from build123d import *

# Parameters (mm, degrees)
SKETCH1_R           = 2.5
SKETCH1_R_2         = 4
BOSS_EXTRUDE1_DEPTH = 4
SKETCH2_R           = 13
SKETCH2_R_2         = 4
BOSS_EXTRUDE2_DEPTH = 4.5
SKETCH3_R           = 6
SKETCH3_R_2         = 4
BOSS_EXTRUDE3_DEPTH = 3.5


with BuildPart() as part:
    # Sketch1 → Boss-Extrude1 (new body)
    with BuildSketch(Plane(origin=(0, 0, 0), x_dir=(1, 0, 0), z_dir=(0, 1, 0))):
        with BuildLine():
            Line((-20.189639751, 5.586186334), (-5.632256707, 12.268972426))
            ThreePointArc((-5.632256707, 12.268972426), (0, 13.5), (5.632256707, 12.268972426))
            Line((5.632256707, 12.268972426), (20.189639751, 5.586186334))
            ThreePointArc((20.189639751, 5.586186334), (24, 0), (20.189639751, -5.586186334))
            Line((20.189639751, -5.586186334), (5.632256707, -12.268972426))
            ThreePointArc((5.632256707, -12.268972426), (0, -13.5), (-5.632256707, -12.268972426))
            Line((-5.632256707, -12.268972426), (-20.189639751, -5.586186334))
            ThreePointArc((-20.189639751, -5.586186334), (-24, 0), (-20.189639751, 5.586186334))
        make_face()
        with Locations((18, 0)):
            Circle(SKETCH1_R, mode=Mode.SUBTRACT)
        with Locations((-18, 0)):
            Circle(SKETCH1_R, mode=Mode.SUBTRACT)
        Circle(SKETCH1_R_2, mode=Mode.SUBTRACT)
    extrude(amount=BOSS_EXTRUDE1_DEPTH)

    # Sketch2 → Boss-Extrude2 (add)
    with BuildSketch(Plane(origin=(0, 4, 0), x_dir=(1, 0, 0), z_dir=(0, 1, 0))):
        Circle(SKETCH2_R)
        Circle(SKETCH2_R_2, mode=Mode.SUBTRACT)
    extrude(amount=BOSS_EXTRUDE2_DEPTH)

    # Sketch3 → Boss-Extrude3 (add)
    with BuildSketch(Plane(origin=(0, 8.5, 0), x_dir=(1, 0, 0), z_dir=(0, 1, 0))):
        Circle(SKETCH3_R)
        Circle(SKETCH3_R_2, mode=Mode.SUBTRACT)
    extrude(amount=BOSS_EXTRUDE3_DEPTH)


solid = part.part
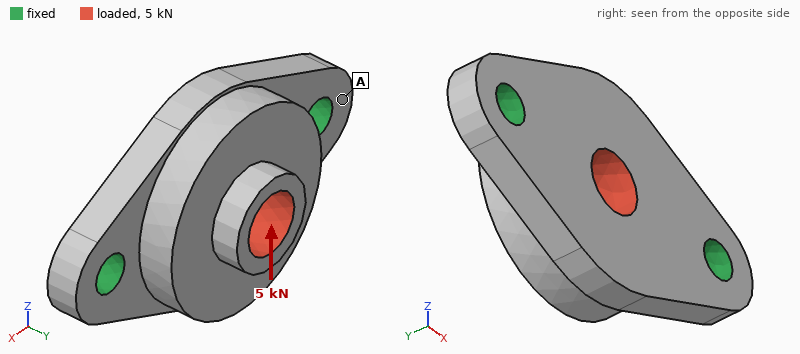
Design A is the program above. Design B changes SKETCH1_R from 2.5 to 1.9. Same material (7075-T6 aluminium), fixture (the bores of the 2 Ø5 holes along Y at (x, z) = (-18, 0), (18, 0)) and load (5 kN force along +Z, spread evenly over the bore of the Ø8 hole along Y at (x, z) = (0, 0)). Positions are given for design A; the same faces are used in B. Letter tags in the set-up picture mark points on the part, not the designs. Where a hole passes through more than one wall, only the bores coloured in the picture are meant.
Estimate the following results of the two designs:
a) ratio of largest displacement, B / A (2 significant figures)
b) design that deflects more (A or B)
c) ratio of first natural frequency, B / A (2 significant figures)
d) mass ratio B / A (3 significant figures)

1.2
B
0.89
1.01
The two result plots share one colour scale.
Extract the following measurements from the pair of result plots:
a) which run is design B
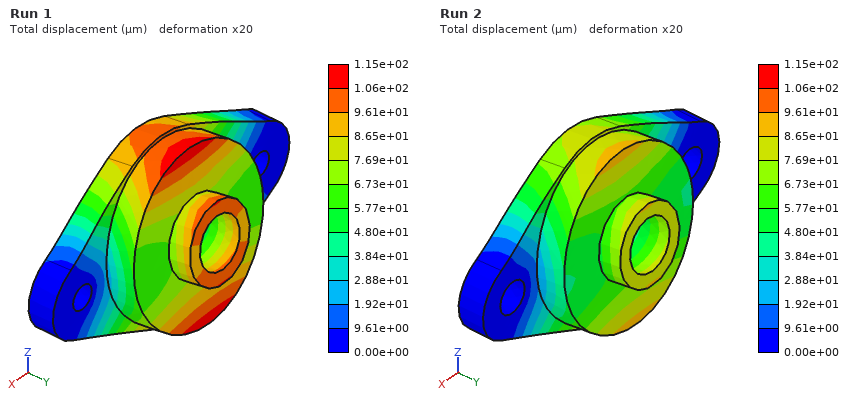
Run 1
